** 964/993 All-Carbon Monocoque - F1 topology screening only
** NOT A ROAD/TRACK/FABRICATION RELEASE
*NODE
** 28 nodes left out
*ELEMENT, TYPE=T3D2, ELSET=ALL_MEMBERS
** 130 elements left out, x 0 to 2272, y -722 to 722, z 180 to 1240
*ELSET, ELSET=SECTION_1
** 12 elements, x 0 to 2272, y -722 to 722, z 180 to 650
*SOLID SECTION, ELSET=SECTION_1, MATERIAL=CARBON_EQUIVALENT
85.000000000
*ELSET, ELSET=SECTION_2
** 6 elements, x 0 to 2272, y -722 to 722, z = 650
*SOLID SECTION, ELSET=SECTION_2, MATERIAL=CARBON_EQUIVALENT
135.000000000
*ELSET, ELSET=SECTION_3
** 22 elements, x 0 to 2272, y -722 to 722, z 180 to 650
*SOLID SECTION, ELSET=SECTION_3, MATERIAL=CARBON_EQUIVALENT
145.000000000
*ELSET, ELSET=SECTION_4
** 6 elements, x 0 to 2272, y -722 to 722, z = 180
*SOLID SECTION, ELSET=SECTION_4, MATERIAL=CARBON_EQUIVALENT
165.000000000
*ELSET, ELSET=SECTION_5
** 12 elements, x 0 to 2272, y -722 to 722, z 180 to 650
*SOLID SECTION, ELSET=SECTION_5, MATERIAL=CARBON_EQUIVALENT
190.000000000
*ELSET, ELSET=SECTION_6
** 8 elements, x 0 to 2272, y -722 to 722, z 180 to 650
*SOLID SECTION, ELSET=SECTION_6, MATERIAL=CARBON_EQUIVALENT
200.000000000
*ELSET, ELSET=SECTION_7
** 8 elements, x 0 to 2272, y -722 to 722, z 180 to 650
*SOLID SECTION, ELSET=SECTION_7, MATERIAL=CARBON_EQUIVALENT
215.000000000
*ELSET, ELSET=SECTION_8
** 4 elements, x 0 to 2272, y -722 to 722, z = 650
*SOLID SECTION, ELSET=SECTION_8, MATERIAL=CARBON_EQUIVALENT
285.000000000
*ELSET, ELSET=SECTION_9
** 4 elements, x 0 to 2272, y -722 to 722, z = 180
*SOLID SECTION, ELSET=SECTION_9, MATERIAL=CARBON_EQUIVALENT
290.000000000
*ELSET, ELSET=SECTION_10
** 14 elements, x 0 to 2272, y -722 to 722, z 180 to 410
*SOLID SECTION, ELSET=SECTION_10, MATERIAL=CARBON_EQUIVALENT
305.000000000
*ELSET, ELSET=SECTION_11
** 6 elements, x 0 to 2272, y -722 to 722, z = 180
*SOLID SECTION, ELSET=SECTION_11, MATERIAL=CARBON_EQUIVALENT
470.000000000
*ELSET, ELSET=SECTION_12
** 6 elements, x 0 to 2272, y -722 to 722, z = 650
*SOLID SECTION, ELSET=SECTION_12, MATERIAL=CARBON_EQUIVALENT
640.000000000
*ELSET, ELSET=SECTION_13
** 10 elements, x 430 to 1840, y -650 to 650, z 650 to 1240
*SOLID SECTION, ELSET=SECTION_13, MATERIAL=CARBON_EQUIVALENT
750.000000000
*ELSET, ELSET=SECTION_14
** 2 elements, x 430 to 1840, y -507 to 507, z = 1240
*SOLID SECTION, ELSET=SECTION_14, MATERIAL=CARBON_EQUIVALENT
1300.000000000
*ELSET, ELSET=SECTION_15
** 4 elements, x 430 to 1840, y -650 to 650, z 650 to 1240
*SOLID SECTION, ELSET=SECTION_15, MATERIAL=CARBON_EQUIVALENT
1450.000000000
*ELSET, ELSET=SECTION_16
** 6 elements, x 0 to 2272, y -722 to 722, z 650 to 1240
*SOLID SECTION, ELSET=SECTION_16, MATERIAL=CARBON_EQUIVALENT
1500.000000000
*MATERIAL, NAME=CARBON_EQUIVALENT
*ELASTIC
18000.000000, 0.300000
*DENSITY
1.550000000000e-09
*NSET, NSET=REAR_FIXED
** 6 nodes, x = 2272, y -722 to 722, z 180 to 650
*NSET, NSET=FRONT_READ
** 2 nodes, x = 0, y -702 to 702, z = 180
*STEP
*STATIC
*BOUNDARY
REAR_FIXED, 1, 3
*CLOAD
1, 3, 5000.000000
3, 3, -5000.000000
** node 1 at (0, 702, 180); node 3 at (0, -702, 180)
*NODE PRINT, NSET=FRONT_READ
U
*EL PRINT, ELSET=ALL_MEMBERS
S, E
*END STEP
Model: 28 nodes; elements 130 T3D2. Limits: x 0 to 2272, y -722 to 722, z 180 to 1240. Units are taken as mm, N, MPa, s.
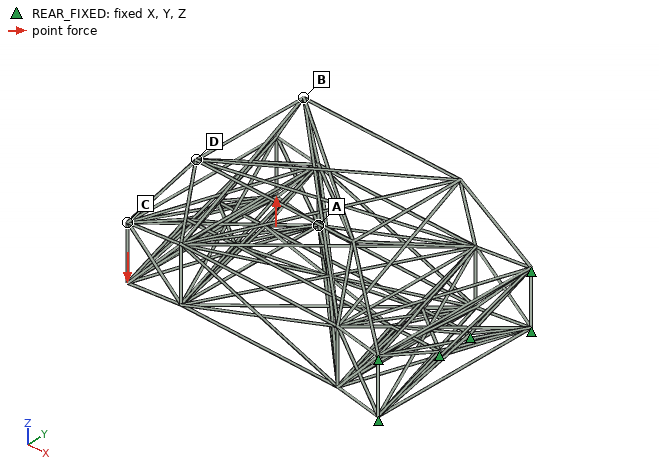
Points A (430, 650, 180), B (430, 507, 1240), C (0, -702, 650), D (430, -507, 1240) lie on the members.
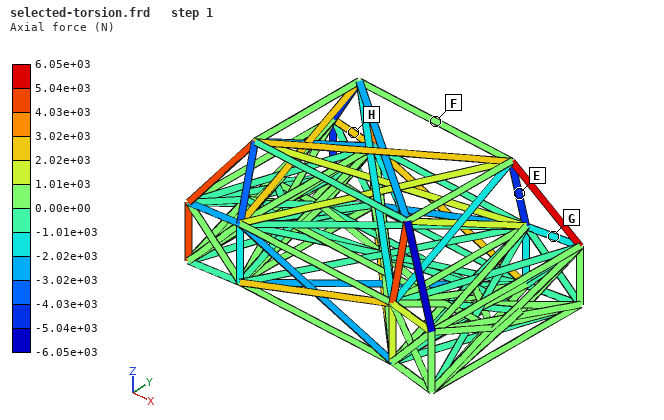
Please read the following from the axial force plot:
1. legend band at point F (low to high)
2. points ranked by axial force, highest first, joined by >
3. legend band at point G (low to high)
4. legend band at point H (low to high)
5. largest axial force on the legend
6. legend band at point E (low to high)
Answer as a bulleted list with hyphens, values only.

- 0.00e+00 to 1.01e+03 N
- H > F > G > E
- -2.02e+03 to -1.01e+03 N
- 2.02e+03 to 3.02e+03 N
- 6.05e+03 N
- -5.04e+03 to -4.03e+03 N
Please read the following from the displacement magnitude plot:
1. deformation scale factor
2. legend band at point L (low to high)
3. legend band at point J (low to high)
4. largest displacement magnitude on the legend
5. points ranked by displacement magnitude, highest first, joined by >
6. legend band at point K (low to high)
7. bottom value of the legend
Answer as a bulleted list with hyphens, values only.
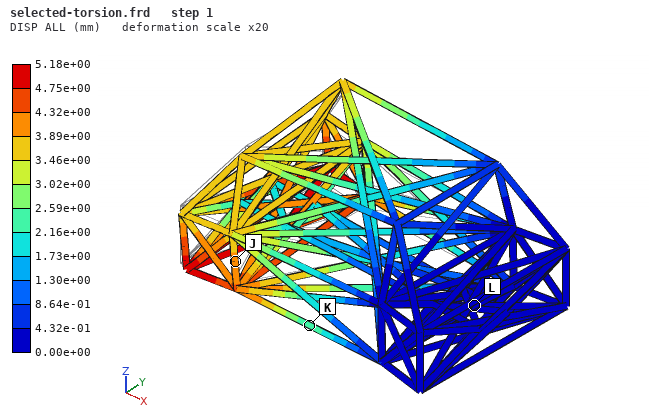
- 20
- 0.00e+00 to 4.32e-01 mm
- 3.89e+00 to 4.32e+00 mm
- 5.18e+00 mm
- J > K > L
- 2.16e+00 to 2.59e+00 mm
- 0.00e+00 mm
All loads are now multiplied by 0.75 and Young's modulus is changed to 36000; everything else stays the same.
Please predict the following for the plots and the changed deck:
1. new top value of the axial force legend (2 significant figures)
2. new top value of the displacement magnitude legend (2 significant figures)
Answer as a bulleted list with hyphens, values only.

- 4500 N
- 1.9 mm
